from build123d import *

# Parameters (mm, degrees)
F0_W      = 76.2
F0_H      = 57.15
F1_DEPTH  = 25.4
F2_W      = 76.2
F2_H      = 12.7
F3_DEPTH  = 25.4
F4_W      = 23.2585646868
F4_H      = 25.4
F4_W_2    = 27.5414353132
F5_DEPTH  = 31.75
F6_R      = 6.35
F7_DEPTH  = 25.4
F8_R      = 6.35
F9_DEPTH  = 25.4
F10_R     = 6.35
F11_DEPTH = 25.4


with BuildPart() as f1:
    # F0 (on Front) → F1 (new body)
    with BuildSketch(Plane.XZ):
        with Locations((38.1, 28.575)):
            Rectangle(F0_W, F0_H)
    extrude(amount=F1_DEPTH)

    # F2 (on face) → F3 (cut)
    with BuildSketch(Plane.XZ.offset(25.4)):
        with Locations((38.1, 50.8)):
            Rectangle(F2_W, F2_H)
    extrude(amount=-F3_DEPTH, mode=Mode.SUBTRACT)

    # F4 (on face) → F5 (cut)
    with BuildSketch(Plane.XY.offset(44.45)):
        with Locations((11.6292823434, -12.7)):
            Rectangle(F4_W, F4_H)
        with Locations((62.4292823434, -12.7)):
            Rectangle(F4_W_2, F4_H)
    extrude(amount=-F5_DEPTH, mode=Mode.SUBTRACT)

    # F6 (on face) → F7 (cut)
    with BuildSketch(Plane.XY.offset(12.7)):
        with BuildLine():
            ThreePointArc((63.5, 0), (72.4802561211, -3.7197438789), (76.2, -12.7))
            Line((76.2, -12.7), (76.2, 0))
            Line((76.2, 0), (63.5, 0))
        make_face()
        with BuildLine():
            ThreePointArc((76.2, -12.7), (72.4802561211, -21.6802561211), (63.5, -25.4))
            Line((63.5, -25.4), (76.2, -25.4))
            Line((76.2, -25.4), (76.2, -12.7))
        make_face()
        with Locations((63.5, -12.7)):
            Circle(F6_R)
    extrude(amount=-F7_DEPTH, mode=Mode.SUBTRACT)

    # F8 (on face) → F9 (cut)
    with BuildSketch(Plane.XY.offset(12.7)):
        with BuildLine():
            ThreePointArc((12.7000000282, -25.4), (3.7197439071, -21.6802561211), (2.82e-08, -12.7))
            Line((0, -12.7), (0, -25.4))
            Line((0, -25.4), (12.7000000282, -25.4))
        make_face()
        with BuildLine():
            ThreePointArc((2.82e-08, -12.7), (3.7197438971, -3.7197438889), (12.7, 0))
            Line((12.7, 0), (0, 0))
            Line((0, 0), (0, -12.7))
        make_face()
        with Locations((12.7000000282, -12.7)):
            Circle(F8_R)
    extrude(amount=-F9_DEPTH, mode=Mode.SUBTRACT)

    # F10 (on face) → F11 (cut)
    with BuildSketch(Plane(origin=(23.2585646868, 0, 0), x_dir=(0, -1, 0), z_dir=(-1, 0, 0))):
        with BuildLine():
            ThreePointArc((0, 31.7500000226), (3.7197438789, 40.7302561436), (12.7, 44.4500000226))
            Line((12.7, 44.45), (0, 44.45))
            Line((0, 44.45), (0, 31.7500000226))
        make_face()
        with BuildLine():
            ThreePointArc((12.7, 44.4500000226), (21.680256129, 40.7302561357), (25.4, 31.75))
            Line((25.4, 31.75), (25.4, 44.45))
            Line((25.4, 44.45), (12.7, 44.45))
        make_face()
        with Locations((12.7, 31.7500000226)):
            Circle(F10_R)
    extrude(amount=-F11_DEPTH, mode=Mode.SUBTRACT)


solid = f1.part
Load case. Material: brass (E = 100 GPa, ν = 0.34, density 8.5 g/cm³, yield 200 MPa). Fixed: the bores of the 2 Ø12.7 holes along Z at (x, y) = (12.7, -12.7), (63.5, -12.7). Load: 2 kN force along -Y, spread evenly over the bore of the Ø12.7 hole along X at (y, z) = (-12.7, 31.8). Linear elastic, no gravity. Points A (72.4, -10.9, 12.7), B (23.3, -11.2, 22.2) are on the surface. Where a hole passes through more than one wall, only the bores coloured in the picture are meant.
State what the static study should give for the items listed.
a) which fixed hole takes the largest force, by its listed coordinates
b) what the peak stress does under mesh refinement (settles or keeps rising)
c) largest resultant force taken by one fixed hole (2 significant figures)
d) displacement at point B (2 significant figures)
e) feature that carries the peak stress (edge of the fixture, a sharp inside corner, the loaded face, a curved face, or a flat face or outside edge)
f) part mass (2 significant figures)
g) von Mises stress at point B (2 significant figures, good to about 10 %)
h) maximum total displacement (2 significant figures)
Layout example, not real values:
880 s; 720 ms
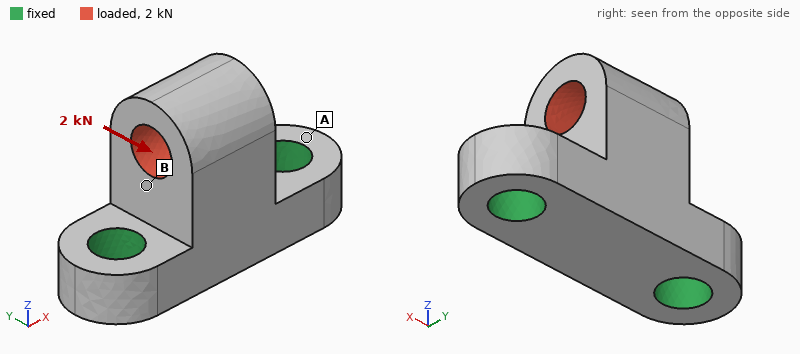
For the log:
(12.7, -12.7); keeps rising; 1.2 kN; 12 µm; edge of the fixture; 300 g; 16 MPa; 30 µm
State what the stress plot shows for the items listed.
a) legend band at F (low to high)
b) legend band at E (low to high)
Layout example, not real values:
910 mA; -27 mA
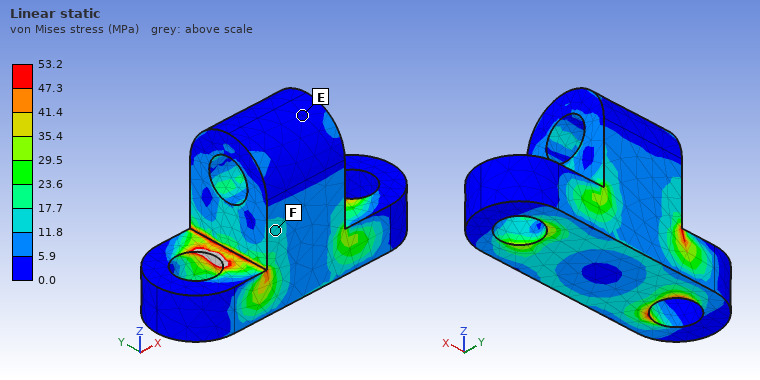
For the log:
11.8 to 17.7 MPa; 0.0 to 5.9 MPa
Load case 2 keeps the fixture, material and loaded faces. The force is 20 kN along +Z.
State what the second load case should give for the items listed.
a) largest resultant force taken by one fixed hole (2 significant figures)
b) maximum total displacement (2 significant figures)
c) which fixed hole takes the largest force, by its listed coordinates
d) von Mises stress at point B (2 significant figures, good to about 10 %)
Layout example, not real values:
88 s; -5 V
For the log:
11 kN; 34 µm; (12.7, -12.7); 29 MPa
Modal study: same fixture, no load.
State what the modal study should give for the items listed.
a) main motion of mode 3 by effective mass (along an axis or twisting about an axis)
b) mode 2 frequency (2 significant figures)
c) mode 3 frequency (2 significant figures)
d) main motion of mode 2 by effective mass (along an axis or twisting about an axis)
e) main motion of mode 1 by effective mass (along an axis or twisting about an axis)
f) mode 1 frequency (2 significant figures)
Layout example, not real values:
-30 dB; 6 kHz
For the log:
along Z; 8000 Hz; 12 kHz; along X; along Y; 4700 Hz
